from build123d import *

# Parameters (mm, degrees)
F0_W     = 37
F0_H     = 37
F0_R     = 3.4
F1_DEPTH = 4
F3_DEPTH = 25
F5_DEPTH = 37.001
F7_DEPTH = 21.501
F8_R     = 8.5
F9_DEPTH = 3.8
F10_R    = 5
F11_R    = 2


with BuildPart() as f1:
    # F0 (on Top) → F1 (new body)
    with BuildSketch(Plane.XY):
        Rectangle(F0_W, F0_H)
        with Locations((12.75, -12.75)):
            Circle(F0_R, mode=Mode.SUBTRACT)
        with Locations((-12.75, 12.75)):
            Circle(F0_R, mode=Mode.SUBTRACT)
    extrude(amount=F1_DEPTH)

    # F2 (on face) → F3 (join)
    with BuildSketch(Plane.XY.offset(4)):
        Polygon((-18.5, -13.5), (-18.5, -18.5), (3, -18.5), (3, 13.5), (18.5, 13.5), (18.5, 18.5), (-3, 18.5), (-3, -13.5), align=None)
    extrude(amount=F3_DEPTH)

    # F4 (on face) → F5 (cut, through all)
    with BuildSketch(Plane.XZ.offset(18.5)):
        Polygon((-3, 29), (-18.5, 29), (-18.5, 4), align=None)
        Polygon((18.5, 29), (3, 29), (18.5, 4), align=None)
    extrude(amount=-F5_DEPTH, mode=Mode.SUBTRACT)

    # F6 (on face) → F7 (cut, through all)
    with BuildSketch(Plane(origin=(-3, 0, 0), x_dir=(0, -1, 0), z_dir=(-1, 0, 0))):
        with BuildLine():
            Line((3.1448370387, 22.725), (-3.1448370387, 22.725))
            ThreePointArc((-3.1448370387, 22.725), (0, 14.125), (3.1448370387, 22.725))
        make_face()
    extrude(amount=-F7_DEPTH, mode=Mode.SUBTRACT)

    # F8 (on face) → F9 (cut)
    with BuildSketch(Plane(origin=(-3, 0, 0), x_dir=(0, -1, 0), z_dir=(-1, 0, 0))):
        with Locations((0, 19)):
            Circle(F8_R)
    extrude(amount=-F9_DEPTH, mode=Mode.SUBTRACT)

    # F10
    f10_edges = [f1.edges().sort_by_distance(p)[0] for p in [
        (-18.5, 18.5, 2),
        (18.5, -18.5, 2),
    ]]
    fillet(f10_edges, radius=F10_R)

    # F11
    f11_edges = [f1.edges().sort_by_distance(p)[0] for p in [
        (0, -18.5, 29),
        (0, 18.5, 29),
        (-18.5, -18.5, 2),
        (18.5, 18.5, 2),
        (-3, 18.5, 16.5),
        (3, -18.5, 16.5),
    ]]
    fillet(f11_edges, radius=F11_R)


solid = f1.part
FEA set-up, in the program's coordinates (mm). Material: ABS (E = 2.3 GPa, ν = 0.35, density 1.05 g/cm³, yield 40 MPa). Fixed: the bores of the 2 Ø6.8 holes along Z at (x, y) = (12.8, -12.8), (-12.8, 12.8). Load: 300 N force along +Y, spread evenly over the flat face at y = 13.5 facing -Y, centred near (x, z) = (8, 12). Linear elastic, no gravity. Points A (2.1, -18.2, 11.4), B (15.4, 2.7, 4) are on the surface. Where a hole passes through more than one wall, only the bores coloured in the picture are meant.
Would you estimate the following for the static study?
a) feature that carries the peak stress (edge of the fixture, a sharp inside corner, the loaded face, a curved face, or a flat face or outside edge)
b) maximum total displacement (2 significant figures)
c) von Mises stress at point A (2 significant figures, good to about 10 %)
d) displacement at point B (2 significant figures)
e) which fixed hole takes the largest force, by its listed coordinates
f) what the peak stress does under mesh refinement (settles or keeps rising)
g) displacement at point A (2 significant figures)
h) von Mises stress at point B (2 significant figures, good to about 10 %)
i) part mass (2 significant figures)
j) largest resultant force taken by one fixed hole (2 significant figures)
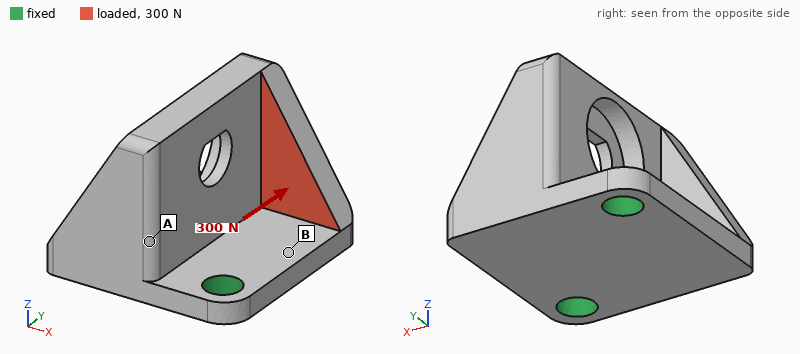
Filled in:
edge of the fixture
0.55 mm
1.9 MPa
0.12 mm
(12.8, -12.8)
keeps rising
0.25 mm
6.3 MPa
12 g
220 N
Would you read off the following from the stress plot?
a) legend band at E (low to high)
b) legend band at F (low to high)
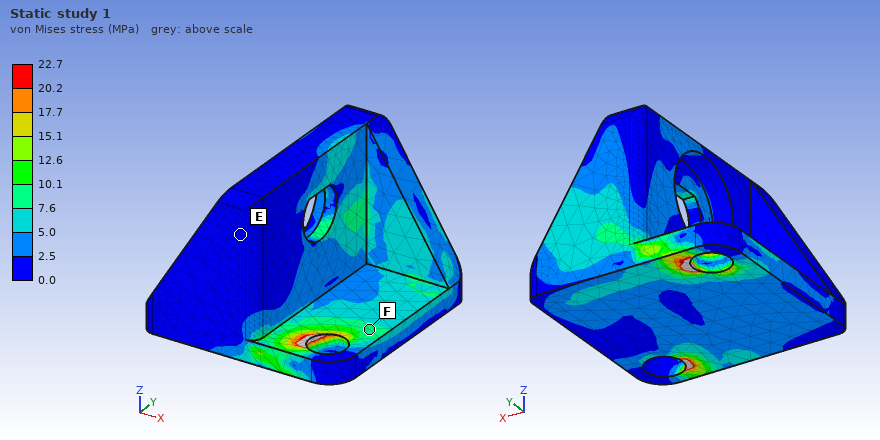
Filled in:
0.0 to 2.5 MPa
7.6 to 10.1 MPa
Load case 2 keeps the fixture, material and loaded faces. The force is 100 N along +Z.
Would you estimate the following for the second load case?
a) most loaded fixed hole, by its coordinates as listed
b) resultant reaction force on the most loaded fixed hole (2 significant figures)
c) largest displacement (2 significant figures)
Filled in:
(-12.8, 12.8)
62 N
0.52 mm
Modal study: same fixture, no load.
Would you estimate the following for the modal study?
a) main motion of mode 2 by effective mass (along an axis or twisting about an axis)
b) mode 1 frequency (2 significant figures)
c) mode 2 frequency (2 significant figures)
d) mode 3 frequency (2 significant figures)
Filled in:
along Z
950 Hz
2000 Hz
2400 Hz
